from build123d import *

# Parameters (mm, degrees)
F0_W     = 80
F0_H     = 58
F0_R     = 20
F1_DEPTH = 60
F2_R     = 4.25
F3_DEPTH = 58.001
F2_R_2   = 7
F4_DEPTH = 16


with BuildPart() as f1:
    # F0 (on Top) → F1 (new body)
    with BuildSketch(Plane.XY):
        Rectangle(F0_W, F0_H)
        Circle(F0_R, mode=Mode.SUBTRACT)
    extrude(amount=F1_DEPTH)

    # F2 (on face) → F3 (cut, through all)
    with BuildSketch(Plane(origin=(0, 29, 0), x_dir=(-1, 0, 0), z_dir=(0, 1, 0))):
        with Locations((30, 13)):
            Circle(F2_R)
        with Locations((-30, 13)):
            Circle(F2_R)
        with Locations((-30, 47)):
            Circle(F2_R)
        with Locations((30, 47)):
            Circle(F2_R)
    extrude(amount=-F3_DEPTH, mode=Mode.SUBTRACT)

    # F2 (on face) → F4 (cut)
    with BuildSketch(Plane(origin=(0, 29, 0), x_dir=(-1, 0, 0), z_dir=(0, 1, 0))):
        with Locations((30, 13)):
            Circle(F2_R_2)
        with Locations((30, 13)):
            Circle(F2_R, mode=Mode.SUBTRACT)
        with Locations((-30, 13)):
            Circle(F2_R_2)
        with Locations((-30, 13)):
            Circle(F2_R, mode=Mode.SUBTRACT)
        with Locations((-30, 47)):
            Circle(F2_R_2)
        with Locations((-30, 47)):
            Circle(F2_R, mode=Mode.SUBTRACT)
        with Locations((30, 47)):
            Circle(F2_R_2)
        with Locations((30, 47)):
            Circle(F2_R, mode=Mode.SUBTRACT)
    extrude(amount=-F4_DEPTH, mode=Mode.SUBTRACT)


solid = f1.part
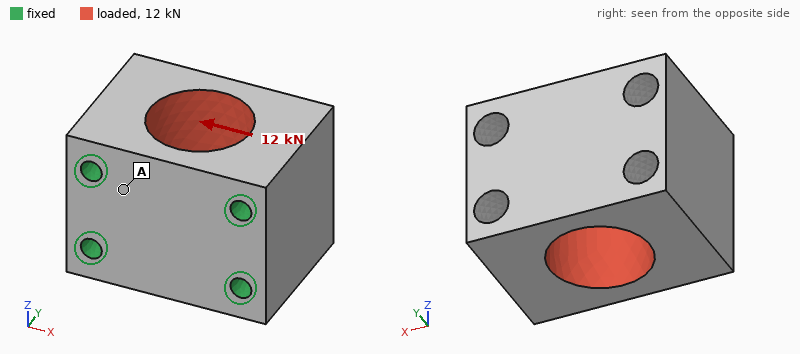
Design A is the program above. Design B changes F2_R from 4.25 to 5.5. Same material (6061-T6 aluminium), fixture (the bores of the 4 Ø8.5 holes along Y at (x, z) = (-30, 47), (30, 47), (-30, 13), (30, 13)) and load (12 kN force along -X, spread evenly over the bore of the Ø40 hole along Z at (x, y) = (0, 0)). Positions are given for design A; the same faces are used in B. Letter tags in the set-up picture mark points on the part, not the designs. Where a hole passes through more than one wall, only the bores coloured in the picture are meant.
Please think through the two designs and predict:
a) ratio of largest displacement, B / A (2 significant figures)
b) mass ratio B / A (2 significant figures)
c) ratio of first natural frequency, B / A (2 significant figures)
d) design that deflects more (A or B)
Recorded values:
0.89
0.96
1.1
A
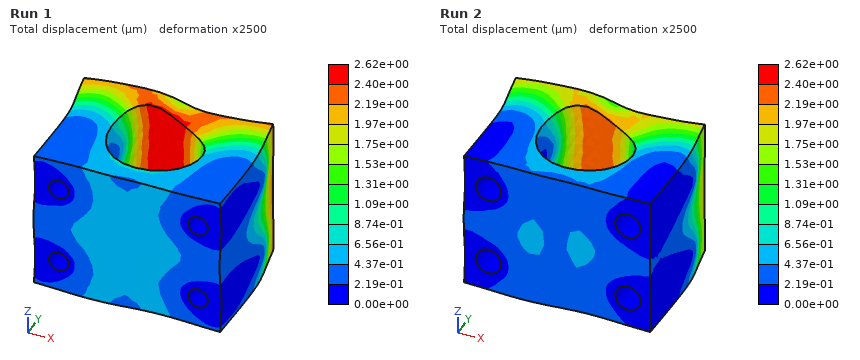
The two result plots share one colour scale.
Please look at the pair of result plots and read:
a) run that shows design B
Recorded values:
Run 2
